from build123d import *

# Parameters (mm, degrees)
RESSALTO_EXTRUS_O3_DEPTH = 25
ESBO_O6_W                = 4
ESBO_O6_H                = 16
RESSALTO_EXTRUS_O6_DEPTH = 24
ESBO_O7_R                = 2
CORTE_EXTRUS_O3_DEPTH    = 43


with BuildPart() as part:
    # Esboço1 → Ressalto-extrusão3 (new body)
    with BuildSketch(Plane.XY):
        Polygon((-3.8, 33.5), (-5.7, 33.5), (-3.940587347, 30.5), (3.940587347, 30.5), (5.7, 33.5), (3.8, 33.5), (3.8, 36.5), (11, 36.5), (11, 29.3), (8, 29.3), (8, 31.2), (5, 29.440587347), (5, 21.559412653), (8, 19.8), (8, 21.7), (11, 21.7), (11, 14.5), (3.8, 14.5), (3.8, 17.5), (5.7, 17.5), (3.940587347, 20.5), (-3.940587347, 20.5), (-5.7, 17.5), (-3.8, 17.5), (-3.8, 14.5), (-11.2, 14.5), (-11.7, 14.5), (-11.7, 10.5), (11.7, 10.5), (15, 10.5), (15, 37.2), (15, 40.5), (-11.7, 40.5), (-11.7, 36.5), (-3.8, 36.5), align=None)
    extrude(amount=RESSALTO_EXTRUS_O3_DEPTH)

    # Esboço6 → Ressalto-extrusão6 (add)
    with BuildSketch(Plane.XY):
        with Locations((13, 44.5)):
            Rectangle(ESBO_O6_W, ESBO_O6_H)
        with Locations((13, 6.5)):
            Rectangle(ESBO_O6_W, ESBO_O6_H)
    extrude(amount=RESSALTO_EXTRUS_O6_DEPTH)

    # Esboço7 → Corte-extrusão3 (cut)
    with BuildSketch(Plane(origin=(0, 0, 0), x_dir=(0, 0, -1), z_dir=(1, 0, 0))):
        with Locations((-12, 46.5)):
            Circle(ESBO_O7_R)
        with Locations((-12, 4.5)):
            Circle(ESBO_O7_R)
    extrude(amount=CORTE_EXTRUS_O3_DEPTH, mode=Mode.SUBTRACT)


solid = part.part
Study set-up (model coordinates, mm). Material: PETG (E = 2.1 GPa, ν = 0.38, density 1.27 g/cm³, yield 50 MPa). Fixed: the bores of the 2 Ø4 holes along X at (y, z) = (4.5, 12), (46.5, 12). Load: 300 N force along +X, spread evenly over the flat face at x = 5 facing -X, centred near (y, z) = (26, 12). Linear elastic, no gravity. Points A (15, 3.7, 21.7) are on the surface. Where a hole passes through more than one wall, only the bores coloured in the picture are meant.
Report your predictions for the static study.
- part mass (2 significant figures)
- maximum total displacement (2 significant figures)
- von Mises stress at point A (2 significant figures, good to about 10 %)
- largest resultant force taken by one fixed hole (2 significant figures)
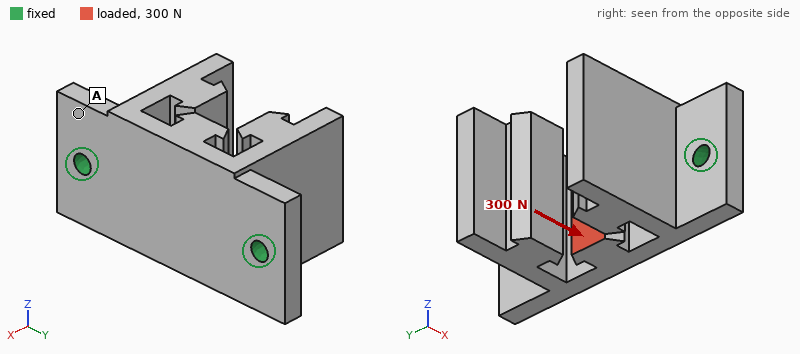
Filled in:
17 g
0.67 mm
5.1 MPa
160 N
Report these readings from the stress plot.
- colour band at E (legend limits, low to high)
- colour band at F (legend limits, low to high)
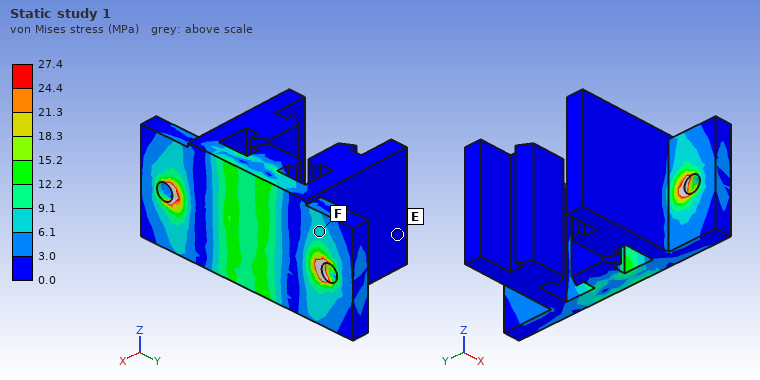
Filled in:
0.0 to 3.0 MPa
6.1 to 9.1 MPa
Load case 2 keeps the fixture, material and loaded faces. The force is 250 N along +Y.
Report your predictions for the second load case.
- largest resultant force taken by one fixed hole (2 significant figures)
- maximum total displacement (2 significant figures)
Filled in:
140 N
0.14 mm
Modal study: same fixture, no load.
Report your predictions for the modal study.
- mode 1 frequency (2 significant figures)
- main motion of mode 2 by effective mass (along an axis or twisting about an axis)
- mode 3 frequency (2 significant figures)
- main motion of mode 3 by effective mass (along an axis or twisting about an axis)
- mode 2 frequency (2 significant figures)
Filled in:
860 Hz
along Z
1100 Hz
along Y
1000 Hz
